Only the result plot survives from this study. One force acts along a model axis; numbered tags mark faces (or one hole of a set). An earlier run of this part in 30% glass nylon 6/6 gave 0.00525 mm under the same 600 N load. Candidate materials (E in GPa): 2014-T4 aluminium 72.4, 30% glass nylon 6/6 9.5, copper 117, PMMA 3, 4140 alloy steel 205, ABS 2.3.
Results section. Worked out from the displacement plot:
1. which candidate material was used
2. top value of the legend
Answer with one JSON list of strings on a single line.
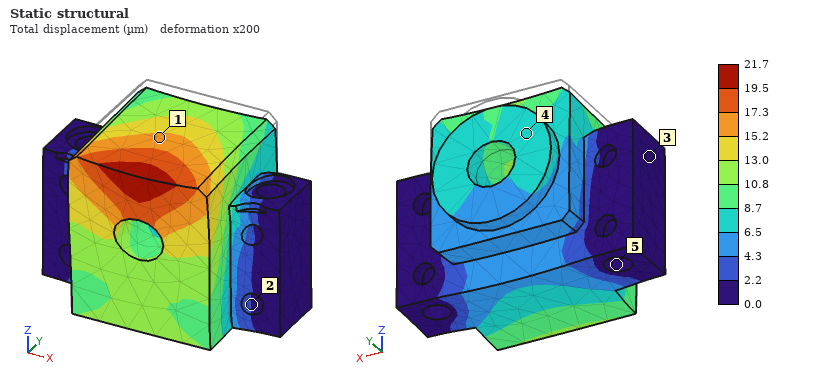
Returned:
["ABS", "21.7 µm"]
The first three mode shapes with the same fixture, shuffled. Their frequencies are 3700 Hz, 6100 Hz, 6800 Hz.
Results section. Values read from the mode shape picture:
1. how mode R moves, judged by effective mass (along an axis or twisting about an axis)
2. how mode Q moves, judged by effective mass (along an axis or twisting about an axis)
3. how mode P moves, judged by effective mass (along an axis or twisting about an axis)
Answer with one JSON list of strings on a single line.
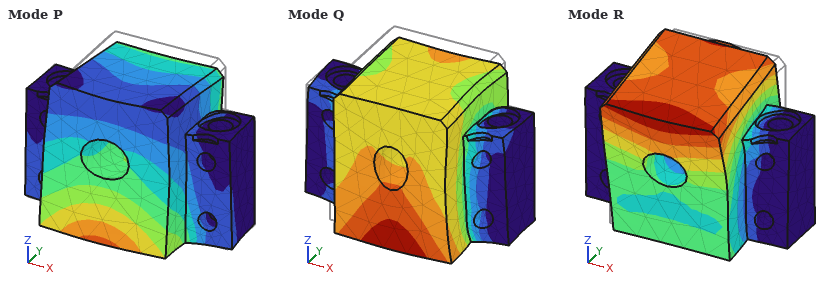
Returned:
["along Y", "along Z", "along Y"]
